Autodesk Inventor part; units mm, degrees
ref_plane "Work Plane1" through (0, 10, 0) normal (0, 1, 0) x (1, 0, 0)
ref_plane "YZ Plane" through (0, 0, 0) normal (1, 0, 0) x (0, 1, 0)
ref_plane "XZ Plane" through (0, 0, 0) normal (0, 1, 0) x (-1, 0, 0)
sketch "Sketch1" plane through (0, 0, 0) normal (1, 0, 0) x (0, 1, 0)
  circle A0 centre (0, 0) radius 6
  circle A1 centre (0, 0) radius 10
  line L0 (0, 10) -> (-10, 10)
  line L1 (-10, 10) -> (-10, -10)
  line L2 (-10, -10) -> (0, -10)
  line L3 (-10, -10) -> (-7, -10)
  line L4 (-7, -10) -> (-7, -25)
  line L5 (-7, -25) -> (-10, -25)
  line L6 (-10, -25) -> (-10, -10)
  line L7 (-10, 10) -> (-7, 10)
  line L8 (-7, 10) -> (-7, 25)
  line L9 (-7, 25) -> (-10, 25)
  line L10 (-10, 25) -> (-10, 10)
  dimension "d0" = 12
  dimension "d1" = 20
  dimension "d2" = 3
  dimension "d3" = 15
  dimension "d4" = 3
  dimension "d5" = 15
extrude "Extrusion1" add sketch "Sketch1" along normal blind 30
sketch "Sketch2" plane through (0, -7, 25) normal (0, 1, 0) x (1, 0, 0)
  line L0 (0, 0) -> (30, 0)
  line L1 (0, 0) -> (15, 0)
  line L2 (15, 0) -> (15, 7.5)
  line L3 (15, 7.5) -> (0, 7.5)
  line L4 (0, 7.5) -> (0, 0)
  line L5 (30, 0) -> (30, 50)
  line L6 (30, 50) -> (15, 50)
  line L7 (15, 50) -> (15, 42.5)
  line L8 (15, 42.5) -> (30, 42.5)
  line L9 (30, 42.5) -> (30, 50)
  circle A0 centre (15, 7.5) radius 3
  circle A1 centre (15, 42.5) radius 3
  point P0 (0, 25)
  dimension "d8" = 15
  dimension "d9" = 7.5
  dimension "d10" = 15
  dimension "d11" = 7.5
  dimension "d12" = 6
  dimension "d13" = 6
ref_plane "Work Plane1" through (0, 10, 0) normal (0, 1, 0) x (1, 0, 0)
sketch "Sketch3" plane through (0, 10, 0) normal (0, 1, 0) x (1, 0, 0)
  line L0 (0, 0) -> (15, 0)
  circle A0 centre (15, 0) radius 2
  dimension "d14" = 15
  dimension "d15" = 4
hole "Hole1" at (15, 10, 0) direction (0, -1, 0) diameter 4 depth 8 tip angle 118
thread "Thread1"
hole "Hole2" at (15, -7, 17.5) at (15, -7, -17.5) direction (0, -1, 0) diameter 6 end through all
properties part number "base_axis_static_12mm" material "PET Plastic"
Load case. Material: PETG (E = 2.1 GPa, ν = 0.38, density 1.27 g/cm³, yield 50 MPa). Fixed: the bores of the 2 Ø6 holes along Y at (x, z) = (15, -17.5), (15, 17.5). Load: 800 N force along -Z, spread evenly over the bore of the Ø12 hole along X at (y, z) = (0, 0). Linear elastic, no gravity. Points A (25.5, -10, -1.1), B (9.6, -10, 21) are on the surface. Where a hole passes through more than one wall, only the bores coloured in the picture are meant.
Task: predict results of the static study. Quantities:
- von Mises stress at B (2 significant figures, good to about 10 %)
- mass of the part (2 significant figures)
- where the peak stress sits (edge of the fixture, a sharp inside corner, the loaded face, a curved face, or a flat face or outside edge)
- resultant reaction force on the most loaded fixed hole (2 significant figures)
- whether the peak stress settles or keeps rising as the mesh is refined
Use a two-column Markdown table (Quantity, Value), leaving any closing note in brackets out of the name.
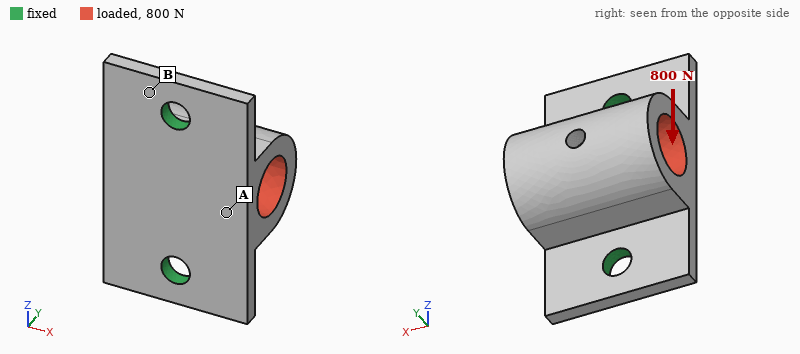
| Quantity | Value |
|---|---|
| von Mises stress at B | 6.5 MPa |
| mass of the part | 12 g |
| where the peak stress sits | edge of the fixture |
| resultant reaction force on the most loaded fixed hole | 470 N |
| whether the peak stress settles or keeps rising as the mesh is refined | keeps rising |
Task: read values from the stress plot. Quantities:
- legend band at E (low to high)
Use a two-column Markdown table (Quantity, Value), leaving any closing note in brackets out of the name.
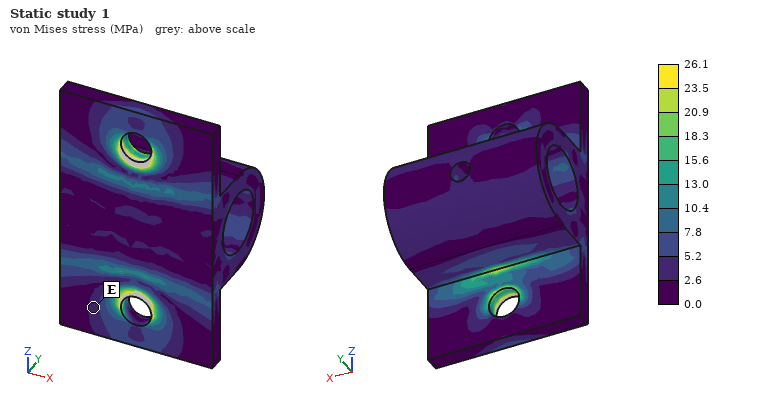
| Quantity | Value |
|---|---|
| legend band at E | 2.6 to 5.2 MPa |
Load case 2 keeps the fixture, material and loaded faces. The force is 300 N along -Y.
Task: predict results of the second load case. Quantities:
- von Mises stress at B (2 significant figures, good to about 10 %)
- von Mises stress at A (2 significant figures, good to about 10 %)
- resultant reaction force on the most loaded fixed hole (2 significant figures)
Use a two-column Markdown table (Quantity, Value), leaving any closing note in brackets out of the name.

| Quantity | Value |
|---|---|
| von Mises stress at B | 2.9 MPa |
| von Mises stress at A | 2.5 MPa |
| resultant reaction force on the most loaded fixed hole | 160 N |
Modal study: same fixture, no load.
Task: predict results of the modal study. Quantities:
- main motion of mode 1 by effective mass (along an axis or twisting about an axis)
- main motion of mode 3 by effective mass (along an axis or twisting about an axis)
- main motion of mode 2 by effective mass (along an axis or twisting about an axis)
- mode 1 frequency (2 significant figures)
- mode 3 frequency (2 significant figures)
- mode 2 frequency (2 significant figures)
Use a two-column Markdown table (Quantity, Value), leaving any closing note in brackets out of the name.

| Quantity | Value |
|---|---|
| main motion of mode 1 by effective mass | along X |
| main motion of mode 3 by effective mass | along Z |
| main motion of mode 2 by effective mass | along Y |
| mode 1 frequency | 1200 Hz |
| mode 3 frequency | 3100 Hz |
| mode 2 frequency | 2800 Hz |
